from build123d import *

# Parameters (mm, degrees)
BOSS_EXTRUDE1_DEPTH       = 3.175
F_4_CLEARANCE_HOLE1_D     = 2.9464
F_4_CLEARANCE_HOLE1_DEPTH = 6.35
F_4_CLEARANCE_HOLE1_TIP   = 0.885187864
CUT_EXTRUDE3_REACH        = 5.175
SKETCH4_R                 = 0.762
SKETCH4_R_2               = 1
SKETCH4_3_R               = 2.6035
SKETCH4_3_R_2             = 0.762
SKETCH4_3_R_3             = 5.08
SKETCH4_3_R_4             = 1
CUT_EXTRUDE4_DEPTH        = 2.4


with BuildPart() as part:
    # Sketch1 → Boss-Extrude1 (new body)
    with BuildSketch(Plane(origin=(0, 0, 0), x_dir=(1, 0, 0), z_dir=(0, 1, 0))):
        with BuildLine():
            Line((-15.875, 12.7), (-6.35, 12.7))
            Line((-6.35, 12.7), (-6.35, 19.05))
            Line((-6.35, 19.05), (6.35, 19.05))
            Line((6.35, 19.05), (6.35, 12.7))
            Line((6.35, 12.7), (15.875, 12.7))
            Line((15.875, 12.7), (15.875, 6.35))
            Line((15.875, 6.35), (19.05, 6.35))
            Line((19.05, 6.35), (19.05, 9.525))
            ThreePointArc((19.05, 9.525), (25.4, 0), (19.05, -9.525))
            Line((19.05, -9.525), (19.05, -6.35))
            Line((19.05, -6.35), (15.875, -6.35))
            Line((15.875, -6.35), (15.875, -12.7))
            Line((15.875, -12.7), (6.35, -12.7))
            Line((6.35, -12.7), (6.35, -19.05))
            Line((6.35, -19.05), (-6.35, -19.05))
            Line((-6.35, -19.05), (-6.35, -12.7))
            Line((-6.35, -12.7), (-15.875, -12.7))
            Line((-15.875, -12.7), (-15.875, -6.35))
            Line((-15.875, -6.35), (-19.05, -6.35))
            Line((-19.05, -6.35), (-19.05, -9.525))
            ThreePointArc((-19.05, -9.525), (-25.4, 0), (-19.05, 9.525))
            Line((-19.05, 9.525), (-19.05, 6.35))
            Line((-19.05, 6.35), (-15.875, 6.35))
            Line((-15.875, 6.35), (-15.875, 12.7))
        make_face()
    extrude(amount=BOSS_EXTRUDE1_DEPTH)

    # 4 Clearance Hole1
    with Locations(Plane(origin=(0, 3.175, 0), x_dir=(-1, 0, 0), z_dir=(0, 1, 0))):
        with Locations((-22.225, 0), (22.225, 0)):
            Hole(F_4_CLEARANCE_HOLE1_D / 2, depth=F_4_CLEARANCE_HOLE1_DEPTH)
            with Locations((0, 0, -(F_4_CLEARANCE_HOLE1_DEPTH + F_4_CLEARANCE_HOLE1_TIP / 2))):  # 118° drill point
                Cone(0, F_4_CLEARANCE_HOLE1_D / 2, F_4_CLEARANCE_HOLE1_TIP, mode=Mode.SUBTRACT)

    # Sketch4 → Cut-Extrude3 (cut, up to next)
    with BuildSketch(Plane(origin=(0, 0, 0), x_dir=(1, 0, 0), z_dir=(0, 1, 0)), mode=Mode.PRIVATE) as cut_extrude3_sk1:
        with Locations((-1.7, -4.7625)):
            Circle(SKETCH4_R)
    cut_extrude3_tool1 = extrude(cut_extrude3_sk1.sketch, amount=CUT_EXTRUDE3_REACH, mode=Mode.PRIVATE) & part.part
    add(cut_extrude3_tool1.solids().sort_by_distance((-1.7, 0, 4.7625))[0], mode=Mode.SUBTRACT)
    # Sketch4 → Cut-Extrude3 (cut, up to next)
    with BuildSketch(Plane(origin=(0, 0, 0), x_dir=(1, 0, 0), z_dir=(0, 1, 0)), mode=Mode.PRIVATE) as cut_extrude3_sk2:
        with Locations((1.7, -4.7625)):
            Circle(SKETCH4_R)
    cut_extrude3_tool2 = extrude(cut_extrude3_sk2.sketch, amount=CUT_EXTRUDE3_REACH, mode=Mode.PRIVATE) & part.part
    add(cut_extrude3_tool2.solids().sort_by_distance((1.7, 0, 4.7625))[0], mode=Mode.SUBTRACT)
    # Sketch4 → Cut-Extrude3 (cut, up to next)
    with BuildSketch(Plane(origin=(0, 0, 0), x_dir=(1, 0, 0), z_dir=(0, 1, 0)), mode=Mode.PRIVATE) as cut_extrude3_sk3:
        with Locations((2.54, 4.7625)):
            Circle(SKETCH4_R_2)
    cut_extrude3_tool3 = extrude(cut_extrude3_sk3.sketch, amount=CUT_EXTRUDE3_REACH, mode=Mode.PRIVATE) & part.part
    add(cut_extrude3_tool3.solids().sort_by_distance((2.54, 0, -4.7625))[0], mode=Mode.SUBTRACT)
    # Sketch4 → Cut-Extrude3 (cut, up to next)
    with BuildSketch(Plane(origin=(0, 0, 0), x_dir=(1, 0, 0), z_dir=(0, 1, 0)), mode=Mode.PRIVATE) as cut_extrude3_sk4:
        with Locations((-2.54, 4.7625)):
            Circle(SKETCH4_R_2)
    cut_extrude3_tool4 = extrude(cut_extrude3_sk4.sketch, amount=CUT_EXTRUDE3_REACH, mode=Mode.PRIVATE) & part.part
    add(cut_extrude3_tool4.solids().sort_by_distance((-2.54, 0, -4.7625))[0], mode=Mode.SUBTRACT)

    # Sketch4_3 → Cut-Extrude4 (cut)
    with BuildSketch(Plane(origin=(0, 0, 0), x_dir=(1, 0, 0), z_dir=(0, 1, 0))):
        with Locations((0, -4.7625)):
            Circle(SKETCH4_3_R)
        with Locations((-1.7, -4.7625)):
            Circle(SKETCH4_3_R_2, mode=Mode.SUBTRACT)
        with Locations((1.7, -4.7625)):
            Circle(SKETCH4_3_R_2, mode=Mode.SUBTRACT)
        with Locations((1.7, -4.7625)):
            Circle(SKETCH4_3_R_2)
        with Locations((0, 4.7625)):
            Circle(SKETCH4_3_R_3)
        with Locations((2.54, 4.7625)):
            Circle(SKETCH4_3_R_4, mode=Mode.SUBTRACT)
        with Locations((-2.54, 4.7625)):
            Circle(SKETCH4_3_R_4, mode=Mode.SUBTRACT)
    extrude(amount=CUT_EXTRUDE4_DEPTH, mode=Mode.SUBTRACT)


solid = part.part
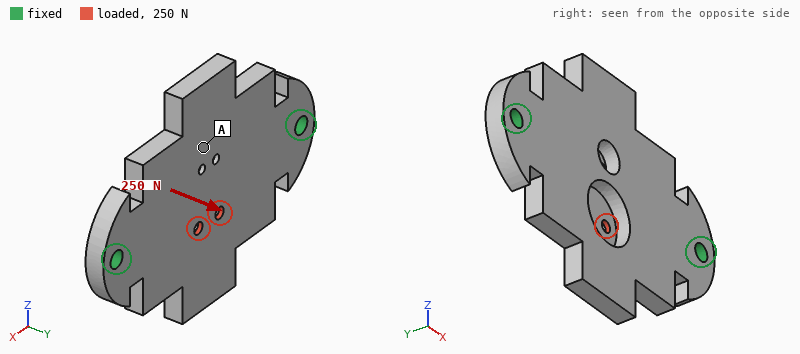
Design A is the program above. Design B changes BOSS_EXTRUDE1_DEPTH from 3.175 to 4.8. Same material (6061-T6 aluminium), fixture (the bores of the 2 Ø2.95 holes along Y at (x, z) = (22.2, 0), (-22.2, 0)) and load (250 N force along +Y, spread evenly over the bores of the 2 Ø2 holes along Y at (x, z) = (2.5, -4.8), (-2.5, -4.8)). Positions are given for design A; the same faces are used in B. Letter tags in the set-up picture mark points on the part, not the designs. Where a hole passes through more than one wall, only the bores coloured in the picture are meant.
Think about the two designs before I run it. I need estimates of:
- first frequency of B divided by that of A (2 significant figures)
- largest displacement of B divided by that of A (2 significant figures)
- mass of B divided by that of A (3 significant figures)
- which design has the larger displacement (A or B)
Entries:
1.4
0.32
1.54
A
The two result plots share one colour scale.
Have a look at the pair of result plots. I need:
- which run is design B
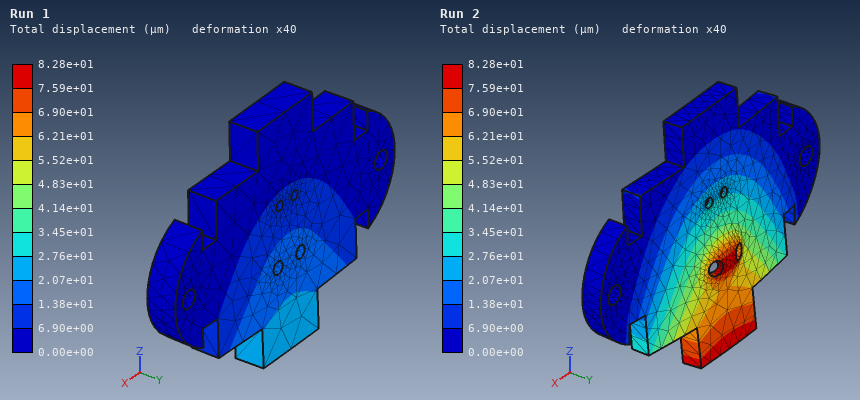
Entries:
Run 1
